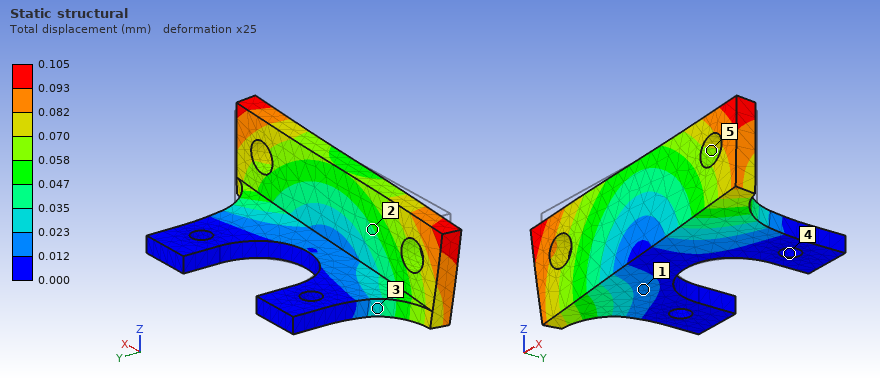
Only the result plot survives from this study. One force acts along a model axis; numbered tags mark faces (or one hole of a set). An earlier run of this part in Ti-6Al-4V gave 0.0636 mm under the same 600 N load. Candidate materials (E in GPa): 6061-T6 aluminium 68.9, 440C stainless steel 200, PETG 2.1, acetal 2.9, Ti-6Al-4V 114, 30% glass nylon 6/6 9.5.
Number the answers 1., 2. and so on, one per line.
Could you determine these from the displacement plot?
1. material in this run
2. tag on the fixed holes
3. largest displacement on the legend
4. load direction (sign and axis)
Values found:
1. 6061-T6 aluminium
2. 4
3. 0.105 mm
4. -X
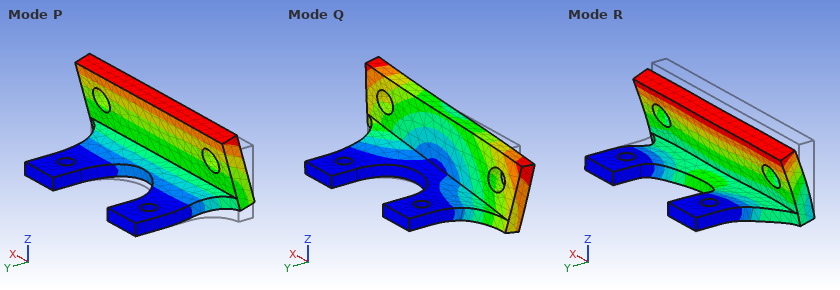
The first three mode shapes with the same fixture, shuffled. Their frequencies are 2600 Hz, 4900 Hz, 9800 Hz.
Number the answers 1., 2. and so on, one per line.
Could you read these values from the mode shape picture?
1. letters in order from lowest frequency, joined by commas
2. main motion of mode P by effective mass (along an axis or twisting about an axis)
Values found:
1. P, Q, R
2. along Z
